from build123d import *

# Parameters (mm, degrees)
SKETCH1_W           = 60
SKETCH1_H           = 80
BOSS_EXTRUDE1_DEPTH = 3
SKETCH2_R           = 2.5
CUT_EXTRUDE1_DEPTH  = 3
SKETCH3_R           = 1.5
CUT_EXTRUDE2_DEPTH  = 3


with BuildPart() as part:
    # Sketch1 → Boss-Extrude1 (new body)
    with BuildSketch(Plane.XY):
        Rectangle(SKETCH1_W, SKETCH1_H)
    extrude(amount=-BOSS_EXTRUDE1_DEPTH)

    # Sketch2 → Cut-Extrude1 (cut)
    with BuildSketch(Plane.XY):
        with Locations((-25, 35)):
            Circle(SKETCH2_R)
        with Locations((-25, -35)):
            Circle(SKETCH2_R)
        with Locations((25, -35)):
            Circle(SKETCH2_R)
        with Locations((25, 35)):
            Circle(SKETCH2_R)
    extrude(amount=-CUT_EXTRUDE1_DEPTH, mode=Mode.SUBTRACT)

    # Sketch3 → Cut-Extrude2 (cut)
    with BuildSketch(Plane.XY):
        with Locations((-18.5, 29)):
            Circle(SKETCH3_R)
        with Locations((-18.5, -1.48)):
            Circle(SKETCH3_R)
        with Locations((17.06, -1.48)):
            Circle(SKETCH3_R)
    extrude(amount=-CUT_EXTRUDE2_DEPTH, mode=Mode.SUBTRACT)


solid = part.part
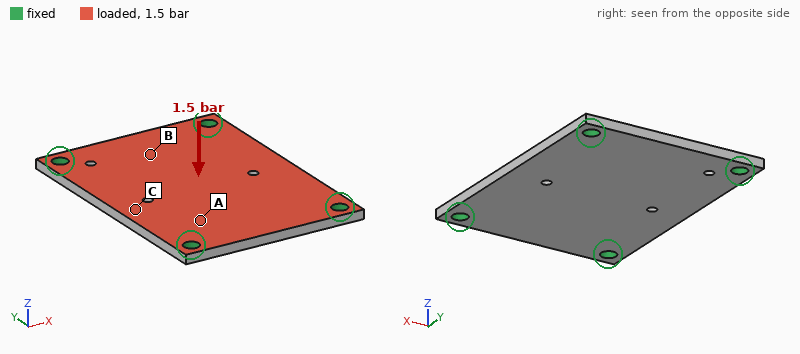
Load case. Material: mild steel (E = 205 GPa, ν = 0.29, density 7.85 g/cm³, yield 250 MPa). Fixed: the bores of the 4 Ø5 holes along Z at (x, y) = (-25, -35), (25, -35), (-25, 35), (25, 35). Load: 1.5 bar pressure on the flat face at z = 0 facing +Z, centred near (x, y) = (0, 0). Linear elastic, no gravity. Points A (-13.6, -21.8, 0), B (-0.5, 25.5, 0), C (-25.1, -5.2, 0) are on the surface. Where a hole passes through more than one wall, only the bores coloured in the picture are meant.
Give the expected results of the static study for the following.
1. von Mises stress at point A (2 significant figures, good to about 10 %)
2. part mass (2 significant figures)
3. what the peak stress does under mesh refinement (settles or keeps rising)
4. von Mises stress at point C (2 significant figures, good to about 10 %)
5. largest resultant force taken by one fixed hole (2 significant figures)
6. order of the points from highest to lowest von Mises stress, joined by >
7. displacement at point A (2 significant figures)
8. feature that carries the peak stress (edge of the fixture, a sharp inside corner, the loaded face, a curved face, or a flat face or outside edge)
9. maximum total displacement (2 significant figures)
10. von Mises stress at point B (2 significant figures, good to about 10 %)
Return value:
7.1 MPa
110 g
keeps rising
23 MPa
180 N
C > B > A
15 µm
edge of the fixture
30 µm
14 MPa
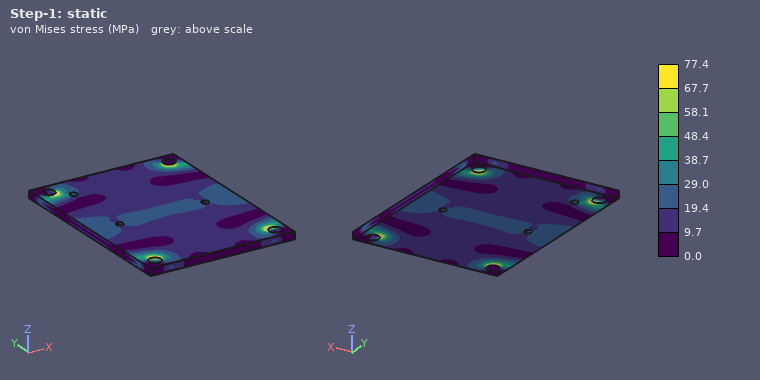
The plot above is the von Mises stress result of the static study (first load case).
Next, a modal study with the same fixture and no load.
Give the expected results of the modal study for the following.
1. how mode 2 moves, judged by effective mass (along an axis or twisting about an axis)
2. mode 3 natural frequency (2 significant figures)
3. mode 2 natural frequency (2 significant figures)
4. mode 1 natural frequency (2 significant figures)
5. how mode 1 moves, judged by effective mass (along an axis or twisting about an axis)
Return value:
twisting about Y
6200 Hz
4200 Hz
2700 Hz
along Z
